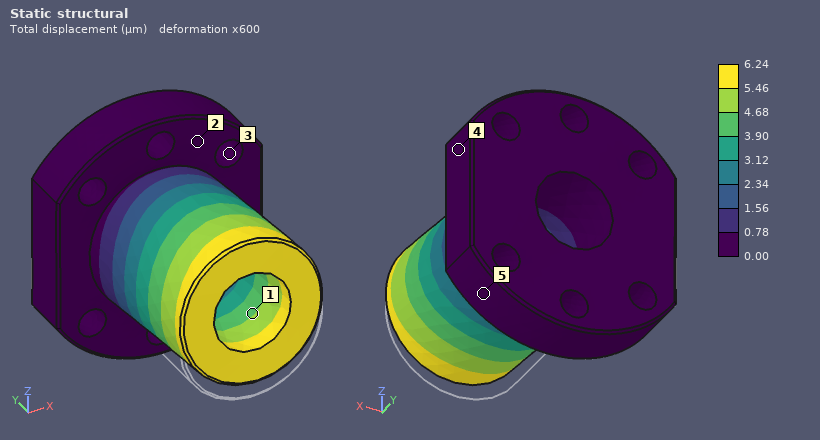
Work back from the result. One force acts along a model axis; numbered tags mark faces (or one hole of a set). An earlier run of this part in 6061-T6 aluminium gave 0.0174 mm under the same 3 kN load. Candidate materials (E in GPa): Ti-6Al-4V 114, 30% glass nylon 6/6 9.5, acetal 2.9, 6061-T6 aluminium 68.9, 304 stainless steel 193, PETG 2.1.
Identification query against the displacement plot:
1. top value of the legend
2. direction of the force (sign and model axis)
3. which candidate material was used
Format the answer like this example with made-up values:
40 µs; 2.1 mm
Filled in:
6.24 µm; +Z; 304 stainless steel
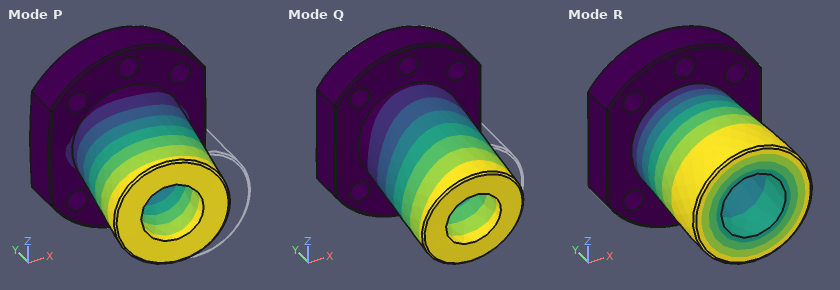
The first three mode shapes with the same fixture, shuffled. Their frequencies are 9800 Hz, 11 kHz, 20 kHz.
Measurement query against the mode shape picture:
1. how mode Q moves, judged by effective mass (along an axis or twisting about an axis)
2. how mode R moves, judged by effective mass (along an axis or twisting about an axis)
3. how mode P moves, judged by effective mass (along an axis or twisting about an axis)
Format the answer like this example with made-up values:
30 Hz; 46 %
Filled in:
along Z; twisting about Y; along X
